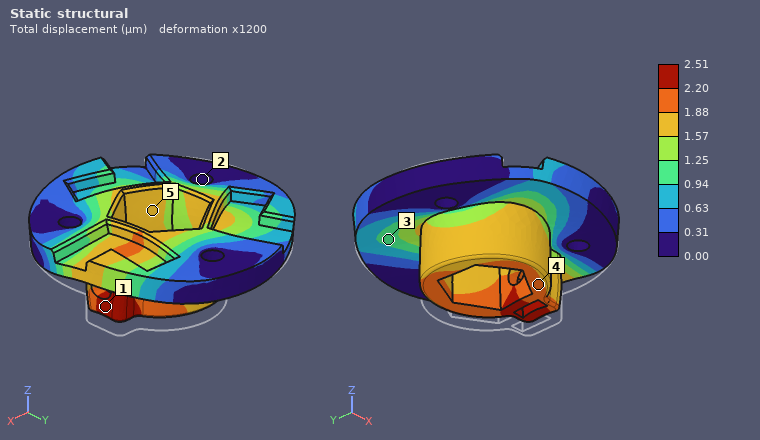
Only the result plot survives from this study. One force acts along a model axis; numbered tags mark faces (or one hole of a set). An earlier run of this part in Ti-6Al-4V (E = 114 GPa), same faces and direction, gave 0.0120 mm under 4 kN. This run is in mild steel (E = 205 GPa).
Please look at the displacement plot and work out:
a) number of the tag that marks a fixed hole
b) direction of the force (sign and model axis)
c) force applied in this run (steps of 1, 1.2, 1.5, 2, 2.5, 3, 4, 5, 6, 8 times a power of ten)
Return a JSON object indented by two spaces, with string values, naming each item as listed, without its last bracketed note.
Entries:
{
  "number of the tag that marks a fixed hole": "2",
  "direction of the force": "+Z",
  "force applied in this run": "1.5 kN"
}
